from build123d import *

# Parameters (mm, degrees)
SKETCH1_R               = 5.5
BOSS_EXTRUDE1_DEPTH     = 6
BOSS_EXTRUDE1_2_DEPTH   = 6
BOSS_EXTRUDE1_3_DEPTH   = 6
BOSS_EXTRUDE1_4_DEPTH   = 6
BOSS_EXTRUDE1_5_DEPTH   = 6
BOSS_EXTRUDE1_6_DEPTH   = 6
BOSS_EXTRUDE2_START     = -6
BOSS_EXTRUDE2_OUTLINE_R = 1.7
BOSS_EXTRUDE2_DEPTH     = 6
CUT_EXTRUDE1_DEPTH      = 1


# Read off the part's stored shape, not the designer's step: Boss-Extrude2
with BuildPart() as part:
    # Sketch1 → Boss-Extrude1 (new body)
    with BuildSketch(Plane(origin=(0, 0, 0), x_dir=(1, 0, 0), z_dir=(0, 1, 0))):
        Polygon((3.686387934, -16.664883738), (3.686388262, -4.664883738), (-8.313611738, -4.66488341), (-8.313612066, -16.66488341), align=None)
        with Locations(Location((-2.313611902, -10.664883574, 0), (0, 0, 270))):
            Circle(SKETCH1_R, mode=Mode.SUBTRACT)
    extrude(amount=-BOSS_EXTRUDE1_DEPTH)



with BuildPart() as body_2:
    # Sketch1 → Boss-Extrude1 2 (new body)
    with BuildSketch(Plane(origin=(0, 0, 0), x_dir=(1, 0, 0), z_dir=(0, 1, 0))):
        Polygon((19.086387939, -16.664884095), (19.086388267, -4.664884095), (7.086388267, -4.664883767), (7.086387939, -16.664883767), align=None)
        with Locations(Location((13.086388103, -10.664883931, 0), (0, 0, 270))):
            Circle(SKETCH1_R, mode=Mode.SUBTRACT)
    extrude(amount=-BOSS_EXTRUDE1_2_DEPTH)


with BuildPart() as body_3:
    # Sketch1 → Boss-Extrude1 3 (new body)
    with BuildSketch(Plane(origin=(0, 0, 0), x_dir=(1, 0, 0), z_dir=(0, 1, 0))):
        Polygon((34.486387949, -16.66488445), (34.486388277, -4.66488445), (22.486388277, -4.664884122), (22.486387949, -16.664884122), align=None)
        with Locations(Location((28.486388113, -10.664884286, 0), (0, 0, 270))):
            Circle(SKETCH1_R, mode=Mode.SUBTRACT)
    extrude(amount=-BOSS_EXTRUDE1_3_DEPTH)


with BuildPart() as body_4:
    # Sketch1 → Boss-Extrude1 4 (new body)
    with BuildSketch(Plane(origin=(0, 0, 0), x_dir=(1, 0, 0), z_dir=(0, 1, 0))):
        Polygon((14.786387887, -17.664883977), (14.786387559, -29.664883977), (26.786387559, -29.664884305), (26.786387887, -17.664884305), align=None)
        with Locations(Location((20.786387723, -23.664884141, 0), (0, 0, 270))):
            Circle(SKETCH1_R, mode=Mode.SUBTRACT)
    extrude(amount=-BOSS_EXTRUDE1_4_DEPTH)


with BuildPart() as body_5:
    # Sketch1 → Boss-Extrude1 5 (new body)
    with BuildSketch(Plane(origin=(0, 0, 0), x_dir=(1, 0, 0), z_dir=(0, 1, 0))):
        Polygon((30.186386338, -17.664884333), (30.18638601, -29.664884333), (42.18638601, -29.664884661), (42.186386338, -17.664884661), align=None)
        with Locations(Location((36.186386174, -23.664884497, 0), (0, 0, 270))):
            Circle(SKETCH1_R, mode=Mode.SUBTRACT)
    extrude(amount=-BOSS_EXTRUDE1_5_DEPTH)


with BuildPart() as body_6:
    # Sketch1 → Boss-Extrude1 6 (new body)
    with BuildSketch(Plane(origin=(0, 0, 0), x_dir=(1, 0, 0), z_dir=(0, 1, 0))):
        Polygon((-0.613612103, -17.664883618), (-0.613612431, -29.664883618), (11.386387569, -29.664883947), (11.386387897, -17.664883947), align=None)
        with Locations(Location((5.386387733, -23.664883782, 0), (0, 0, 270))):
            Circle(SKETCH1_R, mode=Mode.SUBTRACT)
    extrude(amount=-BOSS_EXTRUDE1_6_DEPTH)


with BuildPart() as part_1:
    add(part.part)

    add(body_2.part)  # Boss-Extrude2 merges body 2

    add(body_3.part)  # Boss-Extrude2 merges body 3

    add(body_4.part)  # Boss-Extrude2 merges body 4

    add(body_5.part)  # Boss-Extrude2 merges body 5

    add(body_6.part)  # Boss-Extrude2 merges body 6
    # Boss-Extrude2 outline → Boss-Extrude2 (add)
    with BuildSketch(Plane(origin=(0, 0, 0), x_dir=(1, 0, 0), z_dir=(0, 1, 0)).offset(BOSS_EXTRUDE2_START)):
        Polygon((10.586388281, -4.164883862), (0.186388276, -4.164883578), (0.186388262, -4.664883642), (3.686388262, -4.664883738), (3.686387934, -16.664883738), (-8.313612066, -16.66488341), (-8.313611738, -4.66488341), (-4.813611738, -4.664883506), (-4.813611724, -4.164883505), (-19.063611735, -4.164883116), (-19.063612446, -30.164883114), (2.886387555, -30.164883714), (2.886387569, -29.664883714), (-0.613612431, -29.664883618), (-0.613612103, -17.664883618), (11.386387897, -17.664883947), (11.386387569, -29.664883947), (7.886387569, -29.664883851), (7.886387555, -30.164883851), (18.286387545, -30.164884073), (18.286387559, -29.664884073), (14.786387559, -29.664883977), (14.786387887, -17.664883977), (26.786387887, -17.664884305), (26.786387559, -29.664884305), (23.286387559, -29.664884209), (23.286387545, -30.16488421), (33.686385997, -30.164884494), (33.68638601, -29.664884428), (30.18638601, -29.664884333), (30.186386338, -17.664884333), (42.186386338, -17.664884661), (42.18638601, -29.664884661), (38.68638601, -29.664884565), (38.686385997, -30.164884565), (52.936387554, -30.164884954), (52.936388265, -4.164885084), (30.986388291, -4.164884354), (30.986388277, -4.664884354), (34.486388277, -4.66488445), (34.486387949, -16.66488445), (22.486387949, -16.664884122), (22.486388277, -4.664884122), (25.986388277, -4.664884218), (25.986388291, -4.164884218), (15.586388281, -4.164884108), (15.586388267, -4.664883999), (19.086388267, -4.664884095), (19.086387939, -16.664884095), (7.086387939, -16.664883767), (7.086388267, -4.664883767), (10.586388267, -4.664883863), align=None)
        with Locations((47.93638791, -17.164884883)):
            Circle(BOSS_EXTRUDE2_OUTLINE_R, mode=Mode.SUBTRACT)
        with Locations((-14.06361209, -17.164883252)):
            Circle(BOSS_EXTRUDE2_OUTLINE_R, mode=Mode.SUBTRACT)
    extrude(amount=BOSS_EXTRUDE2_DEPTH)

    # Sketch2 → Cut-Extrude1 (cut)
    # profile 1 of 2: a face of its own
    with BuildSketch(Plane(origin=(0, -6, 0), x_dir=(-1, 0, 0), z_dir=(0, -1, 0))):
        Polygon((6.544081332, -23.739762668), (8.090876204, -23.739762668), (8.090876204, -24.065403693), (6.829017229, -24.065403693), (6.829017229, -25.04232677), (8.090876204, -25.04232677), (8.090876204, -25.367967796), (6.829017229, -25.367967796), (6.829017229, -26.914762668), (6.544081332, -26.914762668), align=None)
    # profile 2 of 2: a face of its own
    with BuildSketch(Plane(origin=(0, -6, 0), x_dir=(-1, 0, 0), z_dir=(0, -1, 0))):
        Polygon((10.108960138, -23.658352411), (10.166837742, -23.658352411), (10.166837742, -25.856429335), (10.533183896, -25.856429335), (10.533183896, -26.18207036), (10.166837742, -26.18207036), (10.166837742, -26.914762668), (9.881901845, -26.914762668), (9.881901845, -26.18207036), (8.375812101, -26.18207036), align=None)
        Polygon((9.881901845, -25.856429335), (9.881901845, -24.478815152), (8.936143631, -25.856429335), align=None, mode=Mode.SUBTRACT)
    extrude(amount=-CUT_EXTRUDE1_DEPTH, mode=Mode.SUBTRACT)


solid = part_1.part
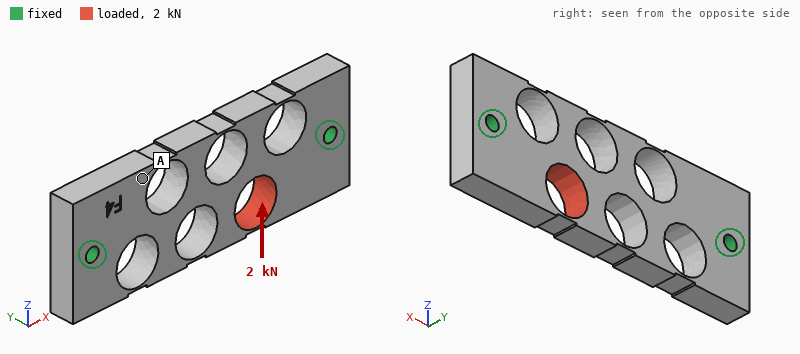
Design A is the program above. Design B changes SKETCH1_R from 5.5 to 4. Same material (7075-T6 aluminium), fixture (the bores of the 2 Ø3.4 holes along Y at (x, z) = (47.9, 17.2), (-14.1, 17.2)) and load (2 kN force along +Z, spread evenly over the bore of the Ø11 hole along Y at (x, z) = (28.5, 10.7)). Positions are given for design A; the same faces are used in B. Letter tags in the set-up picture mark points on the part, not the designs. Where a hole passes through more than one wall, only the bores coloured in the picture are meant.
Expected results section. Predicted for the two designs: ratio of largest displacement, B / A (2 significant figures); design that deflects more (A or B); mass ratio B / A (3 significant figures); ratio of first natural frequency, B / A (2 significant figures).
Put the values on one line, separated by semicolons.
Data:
0.47; A; 1.21; 1.00
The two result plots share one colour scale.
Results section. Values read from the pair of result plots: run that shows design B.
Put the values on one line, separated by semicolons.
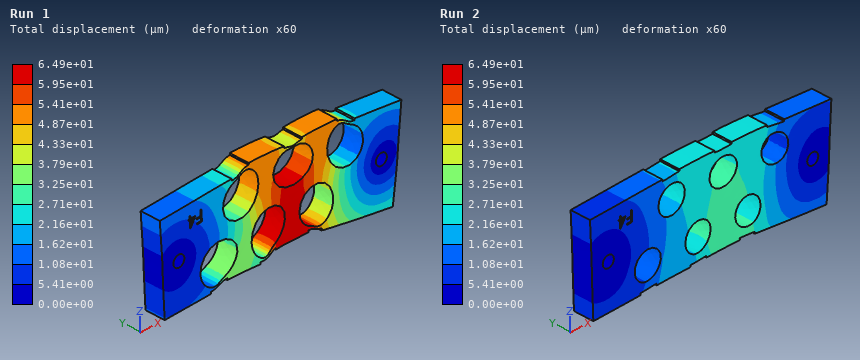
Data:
Run 2
